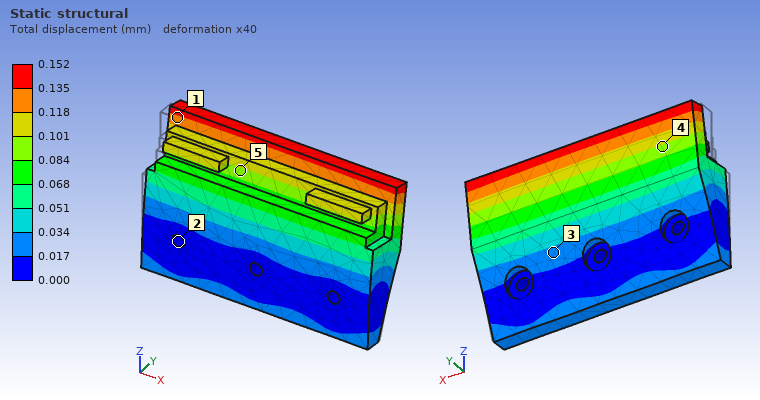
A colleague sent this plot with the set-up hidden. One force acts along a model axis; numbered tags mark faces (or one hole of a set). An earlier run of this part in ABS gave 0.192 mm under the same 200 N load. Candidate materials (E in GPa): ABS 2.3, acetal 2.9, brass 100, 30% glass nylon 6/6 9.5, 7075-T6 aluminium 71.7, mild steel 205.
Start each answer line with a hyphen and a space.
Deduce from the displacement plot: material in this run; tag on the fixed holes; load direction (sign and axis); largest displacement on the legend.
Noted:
- acetal
- 2
- +Y
- 0.152 mm
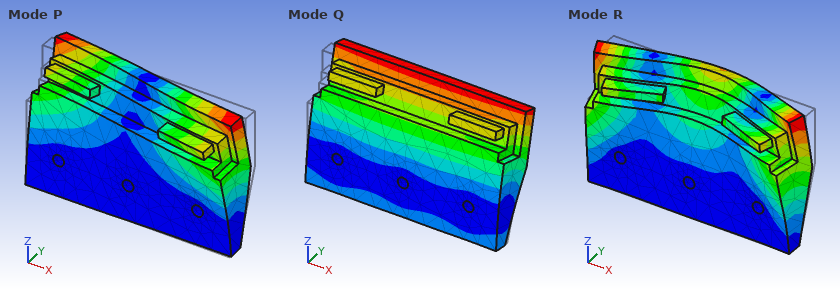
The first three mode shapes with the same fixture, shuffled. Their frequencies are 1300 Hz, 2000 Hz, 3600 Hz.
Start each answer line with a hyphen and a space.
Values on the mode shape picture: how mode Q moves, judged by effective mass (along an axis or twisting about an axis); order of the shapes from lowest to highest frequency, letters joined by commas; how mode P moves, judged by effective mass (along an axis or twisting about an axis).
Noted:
- along Y
- Q, P, R
- twisting about Z
